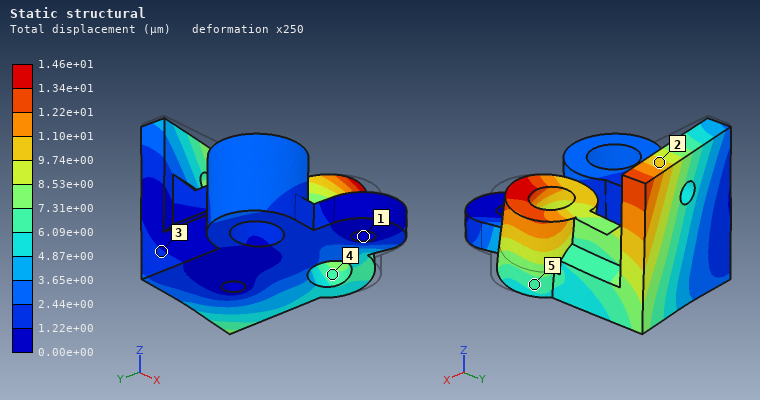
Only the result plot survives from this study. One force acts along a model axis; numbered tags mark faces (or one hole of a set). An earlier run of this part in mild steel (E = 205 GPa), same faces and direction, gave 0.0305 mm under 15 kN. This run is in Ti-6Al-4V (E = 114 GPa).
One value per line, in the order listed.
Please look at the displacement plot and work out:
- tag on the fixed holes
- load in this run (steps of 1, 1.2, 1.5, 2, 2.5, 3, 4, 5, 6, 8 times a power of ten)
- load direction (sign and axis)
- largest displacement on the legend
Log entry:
1
4 kN
+Y
1.46e+01 µm
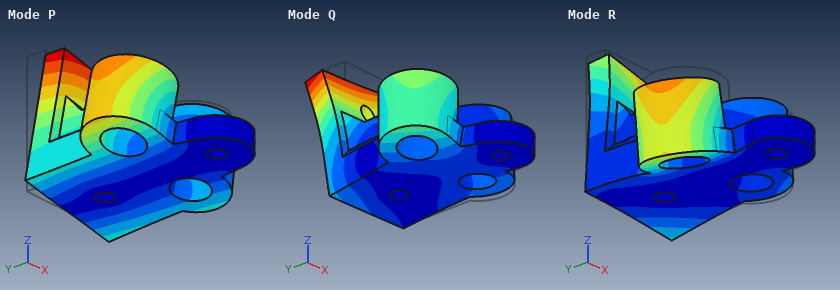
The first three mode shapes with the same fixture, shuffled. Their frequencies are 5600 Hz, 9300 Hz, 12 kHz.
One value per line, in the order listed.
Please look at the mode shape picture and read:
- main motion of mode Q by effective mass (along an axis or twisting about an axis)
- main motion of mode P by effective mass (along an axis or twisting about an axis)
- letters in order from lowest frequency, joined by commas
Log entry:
along Y
along X
P, Q, R
